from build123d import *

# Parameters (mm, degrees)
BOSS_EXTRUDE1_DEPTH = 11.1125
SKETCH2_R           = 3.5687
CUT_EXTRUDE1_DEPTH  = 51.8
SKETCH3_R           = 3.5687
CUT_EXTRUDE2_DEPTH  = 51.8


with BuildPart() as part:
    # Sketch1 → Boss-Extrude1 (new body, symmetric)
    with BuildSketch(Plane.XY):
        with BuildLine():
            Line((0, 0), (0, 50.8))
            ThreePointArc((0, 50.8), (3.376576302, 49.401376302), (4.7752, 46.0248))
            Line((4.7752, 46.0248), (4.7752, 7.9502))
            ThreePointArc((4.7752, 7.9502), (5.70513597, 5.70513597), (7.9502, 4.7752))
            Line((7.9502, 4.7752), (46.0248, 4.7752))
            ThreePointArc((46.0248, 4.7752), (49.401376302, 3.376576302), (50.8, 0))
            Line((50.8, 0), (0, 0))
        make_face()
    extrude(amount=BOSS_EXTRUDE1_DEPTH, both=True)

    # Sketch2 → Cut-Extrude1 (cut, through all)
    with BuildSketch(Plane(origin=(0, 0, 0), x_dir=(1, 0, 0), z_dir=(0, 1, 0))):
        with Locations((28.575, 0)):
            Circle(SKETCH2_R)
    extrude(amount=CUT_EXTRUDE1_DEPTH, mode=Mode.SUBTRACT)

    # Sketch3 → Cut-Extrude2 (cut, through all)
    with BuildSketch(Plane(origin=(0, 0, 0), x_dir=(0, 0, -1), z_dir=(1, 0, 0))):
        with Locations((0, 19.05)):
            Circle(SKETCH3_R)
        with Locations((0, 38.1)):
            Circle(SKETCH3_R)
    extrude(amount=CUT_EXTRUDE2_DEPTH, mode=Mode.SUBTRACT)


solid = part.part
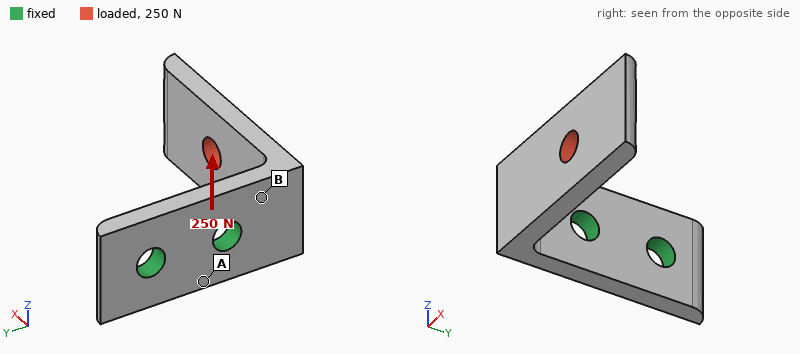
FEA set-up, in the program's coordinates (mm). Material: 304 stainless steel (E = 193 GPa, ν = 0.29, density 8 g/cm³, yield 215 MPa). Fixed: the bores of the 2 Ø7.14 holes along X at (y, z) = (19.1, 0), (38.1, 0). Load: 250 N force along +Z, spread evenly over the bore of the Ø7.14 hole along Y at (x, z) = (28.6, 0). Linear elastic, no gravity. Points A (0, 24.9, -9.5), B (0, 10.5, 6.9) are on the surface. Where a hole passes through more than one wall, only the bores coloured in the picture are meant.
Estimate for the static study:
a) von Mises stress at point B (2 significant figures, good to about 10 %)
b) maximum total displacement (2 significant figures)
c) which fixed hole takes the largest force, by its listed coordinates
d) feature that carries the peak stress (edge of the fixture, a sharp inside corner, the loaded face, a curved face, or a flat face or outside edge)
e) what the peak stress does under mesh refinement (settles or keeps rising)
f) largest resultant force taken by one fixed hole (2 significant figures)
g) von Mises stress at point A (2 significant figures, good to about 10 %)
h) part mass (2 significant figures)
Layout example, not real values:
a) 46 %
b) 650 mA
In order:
a) 37 MPa
b) 64 µm
c) (19.1, 0)
d) edge of the fixture
e) keeps rising
f) 340 N
g) 17 MPa
h) 76 g
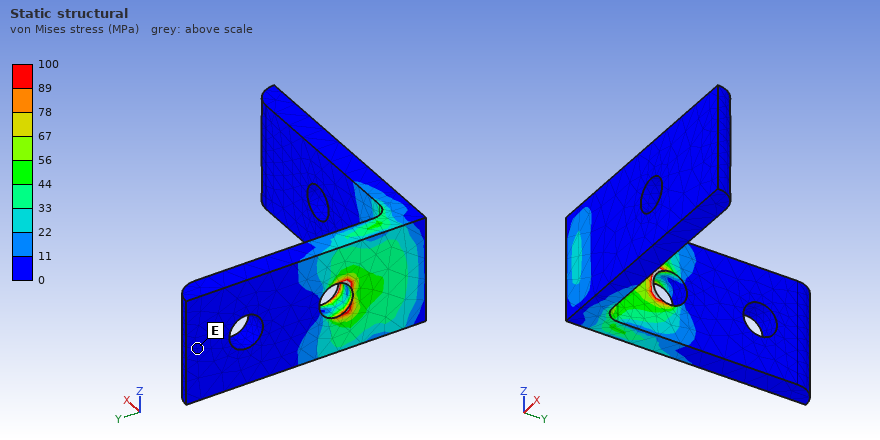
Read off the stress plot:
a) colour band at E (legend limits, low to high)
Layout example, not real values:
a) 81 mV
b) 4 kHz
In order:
a) 0 to 11 MPa
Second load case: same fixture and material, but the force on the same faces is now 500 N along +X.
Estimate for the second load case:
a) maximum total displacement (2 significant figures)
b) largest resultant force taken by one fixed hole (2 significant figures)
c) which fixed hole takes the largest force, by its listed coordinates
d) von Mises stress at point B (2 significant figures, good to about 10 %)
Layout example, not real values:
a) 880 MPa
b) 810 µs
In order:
a) 70 µm
b) 550 N
c) (19.1, 0)
d) 42 MPa
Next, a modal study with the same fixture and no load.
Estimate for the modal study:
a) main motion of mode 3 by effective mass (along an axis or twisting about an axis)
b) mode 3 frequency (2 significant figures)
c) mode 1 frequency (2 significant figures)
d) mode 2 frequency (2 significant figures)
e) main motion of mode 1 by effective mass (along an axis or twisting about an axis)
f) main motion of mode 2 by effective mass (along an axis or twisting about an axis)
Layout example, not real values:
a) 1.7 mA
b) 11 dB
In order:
a) along X
b) 5400 Hz
c) 1200 Hz
d) 2000 Hz
e) along Y
f) along Z
